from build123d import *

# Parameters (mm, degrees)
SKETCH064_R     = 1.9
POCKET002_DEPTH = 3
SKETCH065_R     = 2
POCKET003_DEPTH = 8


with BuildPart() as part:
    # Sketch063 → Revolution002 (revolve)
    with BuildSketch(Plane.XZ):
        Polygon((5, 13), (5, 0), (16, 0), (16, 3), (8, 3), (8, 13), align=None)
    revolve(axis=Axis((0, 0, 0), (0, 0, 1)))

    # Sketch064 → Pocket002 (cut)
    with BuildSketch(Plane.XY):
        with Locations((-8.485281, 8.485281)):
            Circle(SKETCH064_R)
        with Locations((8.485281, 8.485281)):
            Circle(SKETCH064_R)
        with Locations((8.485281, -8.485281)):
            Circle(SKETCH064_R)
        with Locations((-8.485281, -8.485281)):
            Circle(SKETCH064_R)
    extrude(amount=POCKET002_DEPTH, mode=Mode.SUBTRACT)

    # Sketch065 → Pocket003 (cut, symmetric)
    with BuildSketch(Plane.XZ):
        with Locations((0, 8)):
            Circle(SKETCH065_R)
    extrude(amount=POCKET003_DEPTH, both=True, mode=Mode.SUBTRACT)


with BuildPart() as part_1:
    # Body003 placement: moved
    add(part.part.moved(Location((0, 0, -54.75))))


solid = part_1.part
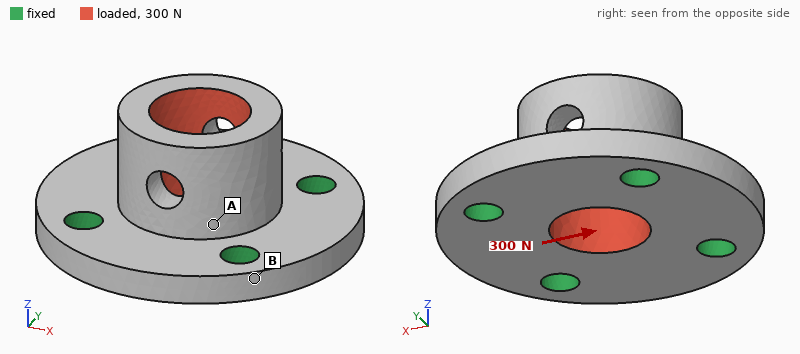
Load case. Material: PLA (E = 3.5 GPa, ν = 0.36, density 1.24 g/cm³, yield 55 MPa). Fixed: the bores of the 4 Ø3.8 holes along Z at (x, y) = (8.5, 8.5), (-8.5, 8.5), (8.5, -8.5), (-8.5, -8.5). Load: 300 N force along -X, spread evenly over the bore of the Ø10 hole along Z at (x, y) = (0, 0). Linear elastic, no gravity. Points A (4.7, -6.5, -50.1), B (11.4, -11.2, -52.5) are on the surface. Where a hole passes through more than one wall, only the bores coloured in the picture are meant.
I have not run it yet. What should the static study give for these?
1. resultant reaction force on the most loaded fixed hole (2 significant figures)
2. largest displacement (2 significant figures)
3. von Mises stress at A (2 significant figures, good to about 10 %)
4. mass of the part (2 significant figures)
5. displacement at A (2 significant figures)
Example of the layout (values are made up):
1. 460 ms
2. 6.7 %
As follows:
1. 91 N
2. 50 µm
3. 3.7 MPa
4. 4.0 g
5. 13 µm
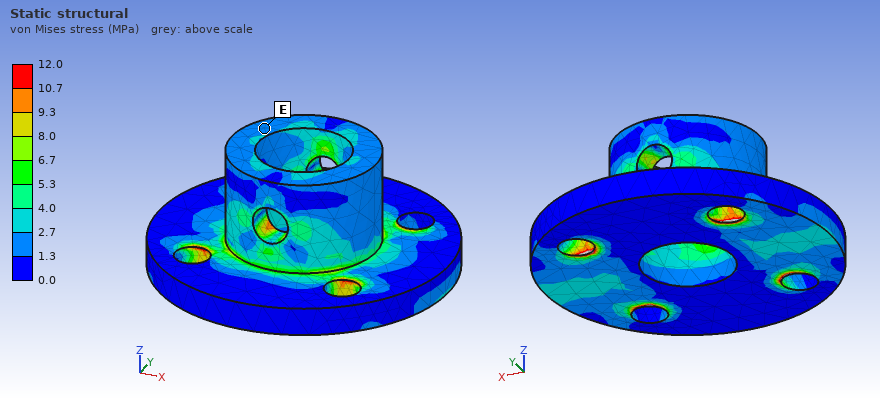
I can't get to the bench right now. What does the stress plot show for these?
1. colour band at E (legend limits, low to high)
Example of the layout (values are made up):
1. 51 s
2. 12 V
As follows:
1. 1.3 to 2.7 MPa
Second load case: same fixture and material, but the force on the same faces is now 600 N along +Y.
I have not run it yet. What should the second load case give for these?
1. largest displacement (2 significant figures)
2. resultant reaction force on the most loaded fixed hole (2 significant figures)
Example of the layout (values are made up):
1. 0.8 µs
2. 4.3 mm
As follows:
1. 86 µm
2. 180 N
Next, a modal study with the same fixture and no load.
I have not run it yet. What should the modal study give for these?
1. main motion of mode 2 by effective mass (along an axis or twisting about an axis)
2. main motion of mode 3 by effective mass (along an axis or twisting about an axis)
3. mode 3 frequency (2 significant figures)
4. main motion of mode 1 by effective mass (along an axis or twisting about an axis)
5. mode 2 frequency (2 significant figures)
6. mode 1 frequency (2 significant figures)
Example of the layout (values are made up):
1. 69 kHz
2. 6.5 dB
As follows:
1. along Y
2. along Z
3. 13 kHz
4. along X
5. 11 kHz
6. 10 kHz
